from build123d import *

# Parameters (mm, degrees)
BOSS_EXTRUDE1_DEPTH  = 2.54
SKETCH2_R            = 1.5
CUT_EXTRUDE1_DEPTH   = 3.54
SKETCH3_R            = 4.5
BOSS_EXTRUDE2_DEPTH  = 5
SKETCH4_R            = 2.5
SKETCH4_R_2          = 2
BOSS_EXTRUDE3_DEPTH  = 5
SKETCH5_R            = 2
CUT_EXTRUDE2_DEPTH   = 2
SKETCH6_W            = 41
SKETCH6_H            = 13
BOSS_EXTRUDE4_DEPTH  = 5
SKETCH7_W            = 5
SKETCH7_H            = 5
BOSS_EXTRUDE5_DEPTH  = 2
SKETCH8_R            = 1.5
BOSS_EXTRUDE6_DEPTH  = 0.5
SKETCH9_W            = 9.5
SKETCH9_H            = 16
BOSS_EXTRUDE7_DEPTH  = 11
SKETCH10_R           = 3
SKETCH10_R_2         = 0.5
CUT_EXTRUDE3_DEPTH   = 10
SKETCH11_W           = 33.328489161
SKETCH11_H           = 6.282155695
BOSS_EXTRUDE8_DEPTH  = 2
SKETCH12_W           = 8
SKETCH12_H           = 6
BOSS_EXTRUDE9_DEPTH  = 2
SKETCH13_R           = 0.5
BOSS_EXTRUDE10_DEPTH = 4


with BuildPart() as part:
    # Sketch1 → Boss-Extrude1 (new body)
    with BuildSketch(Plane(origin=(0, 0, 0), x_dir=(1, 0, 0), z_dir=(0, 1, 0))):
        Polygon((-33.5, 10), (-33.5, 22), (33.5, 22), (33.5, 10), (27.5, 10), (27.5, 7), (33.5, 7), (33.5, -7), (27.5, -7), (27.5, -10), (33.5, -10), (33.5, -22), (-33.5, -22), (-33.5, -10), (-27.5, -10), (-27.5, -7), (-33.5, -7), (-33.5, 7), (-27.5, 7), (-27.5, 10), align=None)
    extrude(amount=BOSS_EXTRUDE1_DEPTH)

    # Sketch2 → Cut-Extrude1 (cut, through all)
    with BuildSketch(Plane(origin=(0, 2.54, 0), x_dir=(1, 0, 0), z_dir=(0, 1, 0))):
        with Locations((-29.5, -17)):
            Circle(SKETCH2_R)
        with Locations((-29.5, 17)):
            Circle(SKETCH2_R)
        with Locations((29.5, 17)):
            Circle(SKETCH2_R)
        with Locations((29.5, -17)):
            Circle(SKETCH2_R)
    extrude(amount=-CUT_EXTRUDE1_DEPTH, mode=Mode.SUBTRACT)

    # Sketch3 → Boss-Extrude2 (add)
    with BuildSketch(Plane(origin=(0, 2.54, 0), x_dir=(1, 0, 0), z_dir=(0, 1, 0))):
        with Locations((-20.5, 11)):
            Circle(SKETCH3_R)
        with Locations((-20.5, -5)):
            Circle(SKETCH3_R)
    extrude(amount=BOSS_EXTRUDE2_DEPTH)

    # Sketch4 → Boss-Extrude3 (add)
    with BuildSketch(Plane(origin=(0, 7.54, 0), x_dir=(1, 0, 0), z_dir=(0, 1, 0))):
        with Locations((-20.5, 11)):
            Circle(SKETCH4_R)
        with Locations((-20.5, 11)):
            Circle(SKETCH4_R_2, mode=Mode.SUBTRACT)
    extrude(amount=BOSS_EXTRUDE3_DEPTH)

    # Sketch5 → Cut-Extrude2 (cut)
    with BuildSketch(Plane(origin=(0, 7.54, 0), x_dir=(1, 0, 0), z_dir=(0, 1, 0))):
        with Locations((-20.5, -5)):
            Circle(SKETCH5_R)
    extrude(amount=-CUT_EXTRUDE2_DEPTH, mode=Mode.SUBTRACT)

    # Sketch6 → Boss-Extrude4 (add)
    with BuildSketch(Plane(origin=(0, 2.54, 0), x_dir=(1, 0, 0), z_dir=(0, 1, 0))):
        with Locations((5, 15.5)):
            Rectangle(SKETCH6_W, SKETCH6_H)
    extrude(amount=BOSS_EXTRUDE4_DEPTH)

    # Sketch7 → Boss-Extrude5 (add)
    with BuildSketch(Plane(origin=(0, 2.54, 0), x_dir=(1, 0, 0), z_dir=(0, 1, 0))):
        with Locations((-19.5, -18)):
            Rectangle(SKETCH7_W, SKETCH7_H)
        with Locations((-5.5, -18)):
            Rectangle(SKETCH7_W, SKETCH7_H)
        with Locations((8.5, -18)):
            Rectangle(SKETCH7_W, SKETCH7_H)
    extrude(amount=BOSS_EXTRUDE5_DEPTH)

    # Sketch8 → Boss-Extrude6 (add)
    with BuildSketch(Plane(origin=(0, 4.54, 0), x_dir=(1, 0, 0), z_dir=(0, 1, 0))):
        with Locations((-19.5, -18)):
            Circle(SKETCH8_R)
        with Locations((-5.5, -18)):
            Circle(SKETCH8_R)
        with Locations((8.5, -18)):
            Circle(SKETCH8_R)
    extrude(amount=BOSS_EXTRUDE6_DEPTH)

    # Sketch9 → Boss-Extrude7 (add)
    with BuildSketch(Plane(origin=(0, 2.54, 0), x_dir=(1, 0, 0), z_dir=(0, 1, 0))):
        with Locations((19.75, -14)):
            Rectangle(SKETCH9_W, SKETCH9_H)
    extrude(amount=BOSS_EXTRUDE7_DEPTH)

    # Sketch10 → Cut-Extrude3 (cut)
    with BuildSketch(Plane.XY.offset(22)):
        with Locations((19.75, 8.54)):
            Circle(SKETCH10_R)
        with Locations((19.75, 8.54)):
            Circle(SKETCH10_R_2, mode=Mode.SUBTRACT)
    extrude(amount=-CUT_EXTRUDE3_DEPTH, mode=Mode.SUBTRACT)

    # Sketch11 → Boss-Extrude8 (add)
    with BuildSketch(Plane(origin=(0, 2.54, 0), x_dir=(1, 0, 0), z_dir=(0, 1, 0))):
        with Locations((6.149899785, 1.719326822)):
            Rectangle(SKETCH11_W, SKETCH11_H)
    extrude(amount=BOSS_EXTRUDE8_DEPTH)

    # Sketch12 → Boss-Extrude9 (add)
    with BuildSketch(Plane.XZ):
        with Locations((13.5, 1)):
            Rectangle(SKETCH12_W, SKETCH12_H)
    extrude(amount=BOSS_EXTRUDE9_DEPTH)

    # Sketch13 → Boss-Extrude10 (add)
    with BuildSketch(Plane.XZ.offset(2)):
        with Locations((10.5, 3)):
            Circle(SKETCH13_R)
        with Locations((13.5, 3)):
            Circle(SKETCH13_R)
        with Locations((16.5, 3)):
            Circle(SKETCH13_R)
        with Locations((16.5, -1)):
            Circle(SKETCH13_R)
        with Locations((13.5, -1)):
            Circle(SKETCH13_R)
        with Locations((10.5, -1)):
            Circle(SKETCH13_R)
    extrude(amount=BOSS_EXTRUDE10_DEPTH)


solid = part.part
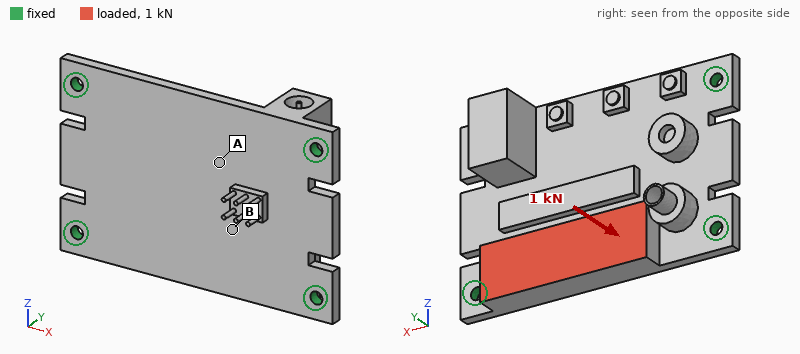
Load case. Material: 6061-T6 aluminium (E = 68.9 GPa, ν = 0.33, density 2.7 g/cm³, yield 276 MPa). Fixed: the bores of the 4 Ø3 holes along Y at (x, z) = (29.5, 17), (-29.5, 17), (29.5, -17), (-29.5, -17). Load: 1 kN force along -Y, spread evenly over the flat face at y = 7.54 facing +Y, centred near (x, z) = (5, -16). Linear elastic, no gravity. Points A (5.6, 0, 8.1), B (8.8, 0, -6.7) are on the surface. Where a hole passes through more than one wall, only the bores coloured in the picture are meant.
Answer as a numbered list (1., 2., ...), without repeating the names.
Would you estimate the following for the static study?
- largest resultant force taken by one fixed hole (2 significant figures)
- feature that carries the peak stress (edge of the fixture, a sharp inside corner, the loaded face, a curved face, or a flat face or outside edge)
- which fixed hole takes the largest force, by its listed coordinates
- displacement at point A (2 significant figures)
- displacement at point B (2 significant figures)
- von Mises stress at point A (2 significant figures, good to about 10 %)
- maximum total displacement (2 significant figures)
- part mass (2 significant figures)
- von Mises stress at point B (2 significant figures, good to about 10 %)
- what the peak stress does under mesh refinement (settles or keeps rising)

1. 820 N
2. edge of the fixture
3. (29.5, -17)
4. 38 µm
5. 52 µm
6. 11 MPa
7. 82 µm
8. 34 g
9. 18 MPa
10. keeps rising
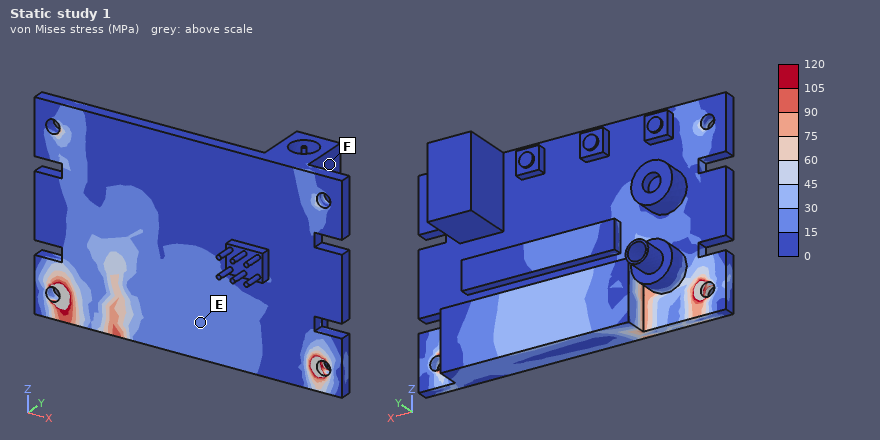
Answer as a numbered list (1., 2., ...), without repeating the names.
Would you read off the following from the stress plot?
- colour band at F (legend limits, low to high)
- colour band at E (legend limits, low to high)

1. 0 to 15 MPa
2. 15 to 30 MPa
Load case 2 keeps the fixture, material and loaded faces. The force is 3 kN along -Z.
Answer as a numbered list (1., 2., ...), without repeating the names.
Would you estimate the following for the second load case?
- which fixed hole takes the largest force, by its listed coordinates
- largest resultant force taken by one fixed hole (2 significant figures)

1. (29.5, -17)
2. 1.2 kN
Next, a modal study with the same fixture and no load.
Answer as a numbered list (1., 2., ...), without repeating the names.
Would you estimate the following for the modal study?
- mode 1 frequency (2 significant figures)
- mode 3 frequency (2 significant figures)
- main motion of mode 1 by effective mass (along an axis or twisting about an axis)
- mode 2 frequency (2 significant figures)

1. 3700 Hz
2. 6800 Hz
3. along Y
4. 5800 Hz
